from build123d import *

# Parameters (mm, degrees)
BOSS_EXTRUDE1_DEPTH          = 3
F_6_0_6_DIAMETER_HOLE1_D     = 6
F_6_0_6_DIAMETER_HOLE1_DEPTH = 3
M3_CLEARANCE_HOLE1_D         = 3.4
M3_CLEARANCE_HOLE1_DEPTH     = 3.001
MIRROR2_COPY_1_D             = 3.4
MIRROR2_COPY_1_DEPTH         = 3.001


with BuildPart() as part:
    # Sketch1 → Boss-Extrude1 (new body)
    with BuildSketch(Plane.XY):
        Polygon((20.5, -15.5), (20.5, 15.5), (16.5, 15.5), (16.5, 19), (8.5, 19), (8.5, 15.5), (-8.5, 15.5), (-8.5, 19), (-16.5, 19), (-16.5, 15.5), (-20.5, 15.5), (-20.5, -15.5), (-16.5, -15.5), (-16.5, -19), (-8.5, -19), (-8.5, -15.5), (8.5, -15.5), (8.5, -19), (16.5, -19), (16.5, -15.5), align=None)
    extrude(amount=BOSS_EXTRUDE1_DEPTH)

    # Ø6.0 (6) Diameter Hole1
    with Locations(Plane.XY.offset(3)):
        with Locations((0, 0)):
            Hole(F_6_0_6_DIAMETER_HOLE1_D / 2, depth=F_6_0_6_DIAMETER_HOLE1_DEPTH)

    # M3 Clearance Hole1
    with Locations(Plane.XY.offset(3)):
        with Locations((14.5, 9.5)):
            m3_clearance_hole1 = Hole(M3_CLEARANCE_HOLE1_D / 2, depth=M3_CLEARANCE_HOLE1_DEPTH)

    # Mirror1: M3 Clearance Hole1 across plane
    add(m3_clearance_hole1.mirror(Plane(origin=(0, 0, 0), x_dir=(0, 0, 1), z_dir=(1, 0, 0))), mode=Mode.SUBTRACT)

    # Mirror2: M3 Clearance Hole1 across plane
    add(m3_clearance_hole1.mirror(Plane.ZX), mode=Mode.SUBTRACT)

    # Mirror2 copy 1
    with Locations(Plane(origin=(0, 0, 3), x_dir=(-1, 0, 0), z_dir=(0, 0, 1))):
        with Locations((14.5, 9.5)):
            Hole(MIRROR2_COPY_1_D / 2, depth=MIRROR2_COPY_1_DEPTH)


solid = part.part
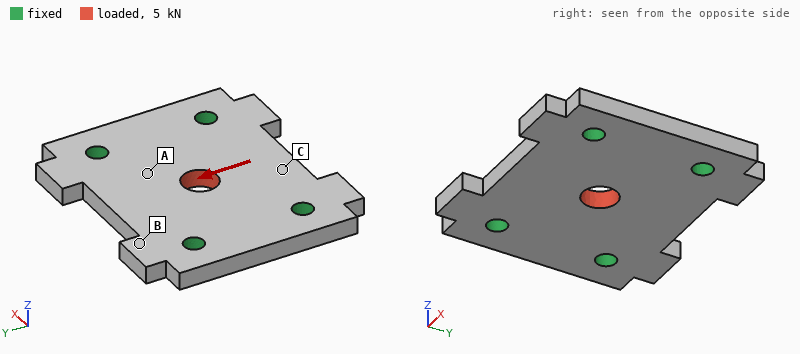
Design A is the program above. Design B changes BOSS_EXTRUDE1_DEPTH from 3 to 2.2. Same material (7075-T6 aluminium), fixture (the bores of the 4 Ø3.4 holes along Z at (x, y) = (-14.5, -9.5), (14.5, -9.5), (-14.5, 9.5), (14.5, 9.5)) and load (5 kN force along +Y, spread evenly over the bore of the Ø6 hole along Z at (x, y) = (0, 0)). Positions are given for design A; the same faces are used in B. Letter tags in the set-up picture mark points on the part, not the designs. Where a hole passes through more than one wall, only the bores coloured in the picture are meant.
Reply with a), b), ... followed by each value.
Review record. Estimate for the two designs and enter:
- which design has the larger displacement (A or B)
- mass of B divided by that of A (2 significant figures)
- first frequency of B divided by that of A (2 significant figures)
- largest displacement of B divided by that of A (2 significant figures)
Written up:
a) B
b) 0.73
c) 0.78
d) 1.4
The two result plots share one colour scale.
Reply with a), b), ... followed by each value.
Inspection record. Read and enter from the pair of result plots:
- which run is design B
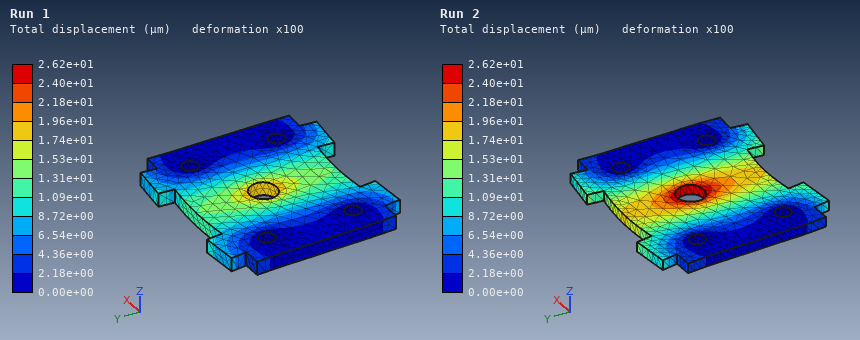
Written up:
a) Run 2
